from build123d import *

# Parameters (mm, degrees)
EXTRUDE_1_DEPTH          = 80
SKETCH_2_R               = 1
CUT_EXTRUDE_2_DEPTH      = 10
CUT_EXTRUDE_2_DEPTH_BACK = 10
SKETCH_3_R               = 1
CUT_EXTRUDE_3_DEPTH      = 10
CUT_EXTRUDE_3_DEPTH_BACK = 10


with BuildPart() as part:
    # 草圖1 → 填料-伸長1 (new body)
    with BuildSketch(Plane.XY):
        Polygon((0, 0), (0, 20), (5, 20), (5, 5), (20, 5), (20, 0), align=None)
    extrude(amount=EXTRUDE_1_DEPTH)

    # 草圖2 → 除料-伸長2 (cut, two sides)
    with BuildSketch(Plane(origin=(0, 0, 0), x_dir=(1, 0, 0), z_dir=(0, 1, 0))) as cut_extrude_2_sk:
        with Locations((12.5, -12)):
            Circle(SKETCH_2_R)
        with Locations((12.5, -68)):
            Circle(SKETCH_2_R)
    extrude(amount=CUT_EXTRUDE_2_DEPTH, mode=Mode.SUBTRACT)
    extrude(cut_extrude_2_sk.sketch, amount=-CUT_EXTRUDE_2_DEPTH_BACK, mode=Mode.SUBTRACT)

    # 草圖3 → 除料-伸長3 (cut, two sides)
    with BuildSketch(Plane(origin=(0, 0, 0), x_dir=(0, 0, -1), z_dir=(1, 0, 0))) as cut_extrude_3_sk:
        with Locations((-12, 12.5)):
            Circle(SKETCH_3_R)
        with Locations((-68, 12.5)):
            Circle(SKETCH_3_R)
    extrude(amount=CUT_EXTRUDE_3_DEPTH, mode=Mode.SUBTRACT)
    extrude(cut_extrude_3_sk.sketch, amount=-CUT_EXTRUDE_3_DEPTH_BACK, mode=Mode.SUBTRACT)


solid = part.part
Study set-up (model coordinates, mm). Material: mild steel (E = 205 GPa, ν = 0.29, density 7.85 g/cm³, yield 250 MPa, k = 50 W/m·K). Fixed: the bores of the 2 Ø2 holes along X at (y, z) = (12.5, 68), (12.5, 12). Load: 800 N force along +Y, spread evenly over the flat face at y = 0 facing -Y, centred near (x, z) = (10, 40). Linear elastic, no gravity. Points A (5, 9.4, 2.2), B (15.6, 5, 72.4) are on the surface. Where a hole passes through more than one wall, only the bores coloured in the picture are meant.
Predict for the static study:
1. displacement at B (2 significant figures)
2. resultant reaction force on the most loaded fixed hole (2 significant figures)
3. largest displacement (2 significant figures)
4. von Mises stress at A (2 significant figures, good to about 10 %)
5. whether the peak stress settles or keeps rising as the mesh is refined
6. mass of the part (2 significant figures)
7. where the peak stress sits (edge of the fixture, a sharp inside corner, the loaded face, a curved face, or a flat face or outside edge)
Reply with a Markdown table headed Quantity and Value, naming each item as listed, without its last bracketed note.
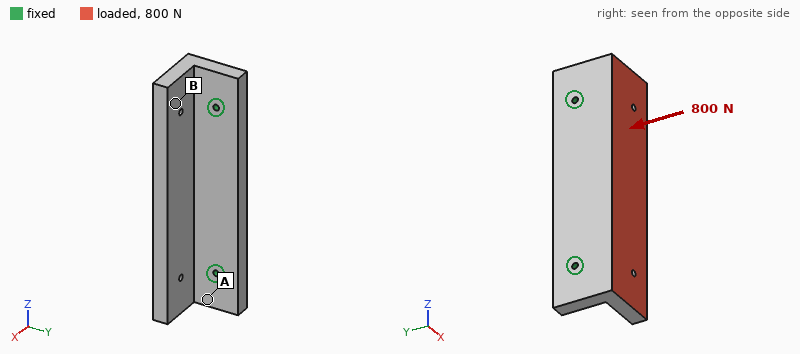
| Quantity | Value |
|---|---|
| displacement at B | 11 µm |
| resultant reaction force on the most loaded fixed hole | 410 N |
| largest displacement | 19 µm |
| von Mises stress at A | 17 MPa |
| whether the peak stress settles or keeps rising as the mesh is refined | keeps rising |
| mass of the part | 110 g |
| where the peak stress sits | edge of the fixture |
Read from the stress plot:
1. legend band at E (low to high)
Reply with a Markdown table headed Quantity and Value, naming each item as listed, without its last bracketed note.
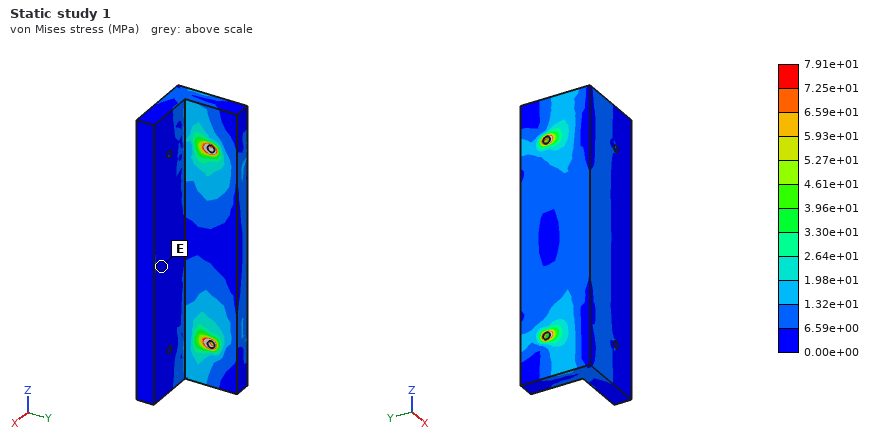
| Quantity | Value |
|---|---|
| legend band at E | 0.00e+00 to 6.59e+00 MPa |
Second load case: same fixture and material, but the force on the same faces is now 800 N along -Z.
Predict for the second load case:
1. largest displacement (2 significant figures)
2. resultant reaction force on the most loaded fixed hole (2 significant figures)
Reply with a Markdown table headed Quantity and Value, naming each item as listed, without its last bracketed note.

| Quantity | Value |
|---|---|
| largest displacement | 2.1 µm |
| resultant reaction force on the most loaded fixed hole | 450 N |
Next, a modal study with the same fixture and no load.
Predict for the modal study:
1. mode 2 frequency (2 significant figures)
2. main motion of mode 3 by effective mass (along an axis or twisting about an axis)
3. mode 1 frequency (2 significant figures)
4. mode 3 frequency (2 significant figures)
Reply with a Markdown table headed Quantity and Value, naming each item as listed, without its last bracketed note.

| Quantity | Value |
|---|---|
| mode 2 frequency | 7300 Hz |
| main motion of mode 3 by effective mass | along X |
| mode 1 frequency | 4400 Hz |
| mode 3 frequency | 9300 Hz |
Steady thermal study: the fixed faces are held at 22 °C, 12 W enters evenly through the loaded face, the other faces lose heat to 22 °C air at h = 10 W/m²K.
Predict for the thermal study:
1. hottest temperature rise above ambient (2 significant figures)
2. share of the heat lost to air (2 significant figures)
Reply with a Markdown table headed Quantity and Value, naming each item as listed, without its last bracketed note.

| Quantity | Value |
|---|---|
| hottest temperature rise above ambient | 19 K |
| share of the heat lost to air | 5.2 % |
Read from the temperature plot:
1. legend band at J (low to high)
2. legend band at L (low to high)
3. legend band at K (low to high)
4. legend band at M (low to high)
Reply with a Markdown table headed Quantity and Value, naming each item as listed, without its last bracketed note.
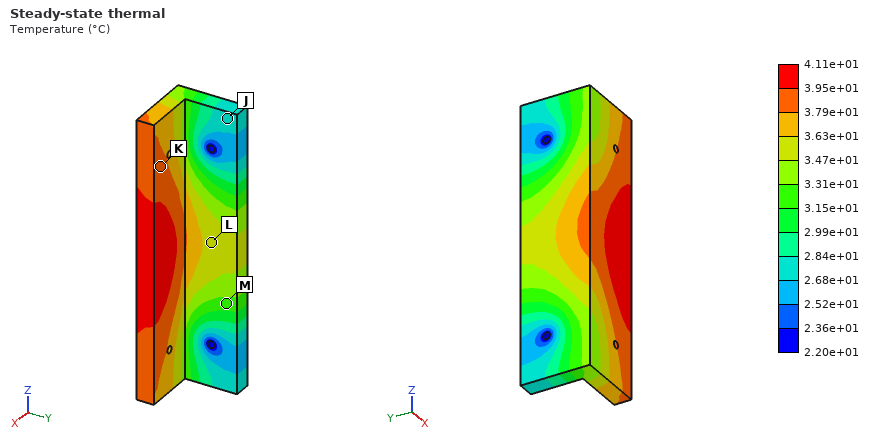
| Quantity | Value |
|---|---|
| legend band at J | 2.68e+01 to 2.84e+01 °C |
| legend band at L | 3.47e+01 to 3.63e+01 °C |
| legend band at K | 3.79e+01 to 3.95e+01 °C |
| legend band at M | 3.15e+01 to 3.31e+01 °C |
